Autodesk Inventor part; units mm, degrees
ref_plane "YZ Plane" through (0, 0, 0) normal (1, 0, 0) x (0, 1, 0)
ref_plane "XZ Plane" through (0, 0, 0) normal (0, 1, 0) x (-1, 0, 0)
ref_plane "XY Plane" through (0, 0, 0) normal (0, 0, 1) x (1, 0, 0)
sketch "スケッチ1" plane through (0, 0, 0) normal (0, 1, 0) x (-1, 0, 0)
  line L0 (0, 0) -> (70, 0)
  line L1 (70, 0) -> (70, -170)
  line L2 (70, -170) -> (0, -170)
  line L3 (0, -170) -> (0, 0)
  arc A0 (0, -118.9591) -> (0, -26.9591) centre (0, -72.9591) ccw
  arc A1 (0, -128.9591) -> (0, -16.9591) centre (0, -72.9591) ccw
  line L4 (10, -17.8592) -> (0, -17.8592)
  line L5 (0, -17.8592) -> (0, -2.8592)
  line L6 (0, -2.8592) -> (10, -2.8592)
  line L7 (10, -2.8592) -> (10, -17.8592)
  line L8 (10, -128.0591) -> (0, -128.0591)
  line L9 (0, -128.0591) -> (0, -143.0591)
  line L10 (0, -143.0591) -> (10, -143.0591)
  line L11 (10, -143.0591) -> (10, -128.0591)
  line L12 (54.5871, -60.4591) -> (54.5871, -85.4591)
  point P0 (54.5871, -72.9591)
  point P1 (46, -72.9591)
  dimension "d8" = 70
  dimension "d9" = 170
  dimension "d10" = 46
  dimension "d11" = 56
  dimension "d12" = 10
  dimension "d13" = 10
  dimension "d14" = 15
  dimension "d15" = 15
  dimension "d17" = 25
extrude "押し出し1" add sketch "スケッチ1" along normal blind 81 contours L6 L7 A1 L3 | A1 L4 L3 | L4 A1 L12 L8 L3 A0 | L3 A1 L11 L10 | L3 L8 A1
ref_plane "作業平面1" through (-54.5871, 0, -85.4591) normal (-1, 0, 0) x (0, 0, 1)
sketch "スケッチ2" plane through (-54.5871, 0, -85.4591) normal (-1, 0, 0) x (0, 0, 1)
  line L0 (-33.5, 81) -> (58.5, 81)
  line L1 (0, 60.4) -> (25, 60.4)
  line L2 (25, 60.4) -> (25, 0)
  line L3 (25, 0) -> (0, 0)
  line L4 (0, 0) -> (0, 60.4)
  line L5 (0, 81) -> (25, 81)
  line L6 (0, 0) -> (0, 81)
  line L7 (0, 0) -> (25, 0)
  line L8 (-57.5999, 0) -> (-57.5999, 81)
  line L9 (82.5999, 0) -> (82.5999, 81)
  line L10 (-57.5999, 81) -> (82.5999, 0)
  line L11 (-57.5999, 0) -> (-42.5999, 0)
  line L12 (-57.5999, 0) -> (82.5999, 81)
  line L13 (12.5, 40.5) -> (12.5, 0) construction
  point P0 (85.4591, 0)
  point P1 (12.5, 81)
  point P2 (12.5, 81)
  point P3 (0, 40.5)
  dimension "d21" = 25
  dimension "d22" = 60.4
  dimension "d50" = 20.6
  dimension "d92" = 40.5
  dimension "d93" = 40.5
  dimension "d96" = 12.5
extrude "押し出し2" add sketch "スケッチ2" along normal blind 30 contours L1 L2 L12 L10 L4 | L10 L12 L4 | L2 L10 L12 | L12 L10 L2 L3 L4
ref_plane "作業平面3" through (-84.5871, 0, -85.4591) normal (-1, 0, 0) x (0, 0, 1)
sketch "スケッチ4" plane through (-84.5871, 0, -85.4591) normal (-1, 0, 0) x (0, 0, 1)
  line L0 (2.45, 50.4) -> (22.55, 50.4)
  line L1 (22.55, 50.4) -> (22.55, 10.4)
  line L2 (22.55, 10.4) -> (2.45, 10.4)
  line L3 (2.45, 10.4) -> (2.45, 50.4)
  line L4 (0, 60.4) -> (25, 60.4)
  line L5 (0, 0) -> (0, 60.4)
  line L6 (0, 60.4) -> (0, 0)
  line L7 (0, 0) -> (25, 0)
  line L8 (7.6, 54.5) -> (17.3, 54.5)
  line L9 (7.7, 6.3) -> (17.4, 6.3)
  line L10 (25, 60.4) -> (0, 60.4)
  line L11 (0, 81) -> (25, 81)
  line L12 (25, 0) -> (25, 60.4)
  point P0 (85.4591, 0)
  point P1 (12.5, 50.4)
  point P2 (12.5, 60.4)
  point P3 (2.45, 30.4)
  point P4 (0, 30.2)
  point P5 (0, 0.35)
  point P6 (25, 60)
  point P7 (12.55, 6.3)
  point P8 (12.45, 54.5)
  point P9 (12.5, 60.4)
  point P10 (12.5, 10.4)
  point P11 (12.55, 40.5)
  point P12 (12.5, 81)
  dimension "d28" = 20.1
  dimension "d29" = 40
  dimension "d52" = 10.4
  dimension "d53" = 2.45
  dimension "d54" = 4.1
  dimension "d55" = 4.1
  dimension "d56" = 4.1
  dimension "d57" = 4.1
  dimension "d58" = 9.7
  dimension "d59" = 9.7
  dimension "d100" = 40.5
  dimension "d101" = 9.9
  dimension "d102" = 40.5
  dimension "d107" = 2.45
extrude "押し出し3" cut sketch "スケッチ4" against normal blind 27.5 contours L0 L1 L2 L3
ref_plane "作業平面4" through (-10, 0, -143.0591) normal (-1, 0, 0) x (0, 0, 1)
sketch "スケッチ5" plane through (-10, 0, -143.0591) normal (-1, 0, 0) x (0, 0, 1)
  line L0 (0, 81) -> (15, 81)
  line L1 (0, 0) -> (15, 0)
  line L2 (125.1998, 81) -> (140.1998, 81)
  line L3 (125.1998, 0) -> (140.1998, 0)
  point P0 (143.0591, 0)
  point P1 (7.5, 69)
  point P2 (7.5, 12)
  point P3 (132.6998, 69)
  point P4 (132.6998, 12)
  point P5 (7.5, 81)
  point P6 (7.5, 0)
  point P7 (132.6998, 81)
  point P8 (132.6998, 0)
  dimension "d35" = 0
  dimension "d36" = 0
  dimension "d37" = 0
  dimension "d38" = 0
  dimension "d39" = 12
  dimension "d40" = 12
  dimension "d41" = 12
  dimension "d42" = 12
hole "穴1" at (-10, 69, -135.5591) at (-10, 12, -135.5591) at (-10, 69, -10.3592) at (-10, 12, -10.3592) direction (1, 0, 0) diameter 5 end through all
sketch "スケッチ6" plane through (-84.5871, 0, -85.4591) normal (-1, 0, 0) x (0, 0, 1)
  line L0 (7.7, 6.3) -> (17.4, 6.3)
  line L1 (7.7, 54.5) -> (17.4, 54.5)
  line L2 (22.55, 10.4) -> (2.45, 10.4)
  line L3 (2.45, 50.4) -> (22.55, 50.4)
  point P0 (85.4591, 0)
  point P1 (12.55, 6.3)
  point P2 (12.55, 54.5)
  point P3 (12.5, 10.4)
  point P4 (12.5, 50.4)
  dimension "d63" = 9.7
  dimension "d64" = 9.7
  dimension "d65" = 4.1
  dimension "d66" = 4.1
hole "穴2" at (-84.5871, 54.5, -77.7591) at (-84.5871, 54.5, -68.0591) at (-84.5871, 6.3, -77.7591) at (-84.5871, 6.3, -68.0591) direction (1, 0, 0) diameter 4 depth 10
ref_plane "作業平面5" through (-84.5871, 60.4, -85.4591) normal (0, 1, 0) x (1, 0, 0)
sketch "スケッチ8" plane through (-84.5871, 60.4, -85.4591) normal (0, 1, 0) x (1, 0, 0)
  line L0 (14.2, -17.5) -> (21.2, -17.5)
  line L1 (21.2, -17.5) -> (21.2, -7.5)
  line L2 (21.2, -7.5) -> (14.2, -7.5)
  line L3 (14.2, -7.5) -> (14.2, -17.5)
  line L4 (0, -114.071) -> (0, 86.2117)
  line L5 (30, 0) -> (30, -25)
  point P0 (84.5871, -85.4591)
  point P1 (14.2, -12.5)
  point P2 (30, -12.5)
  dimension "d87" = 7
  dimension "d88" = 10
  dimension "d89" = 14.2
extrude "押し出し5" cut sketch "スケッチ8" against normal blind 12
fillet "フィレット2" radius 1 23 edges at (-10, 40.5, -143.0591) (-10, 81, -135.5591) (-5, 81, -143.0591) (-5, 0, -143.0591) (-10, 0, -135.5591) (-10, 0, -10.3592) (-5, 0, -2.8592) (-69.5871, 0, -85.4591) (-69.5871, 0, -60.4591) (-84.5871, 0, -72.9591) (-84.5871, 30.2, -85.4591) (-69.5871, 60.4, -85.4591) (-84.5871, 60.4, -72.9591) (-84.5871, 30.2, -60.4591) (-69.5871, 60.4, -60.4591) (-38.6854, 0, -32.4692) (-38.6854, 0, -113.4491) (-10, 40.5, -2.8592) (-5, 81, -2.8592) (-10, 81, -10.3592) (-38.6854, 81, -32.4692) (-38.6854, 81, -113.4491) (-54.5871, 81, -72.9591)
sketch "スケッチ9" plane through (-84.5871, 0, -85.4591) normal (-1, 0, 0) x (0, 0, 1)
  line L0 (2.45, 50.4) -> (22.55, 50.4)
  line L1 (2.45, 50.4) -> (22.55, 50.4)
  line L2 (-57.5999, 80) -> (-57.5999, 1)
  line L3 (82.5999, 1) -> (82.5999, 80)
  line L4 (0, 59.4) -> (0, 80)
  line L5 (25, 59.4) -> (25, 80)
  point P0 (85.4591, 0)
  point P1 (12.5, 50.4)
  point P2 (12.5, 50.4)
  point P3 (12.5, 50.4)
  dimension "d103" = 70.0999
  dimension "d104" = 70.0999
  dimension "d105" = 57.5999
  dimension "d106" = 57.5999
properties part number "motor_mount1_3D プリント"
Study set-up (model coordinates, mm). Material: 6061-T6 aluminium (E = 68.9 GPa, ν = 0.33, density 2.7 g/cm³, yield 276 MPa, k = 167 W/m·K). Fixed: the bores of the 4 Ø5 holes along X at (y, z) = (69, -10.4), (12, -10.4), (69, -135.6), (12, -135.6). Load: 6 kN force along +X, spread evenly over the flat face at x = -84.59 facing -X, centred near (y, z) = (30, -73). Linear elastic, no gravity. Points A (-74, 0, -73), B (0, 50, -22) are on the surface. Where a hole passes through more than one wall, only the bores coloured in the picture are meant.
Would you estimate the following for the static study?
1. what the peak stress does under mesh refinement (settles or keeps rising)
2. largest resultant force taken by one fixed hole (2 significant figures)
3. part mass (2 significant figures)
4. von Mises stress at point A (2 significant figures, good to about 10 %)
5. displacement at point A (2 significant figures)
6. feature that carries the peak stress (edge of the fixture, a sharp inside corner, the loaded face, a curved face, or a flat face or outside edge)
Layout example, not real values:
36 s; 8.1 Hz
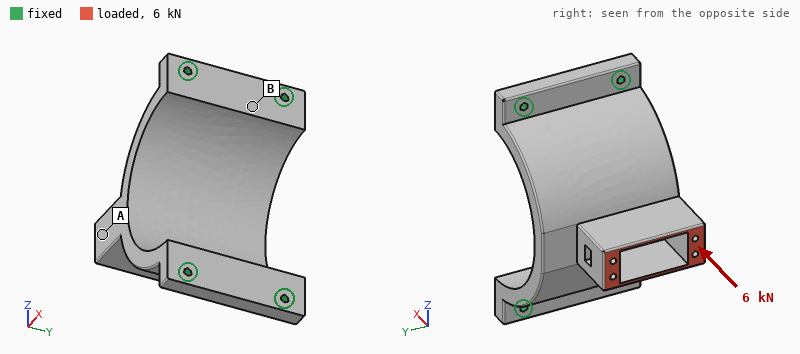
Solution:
keeps rising; 2.7 kN; 460 g; 8.8 MPa; 38 µm; edge of the fixture
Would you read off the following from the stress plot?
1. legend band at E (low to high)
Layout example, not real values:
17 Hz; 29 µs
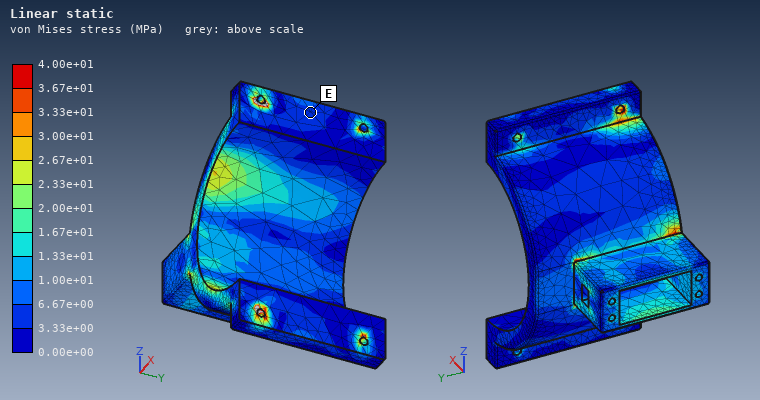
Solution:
3.33e+00 to 6.67e+00 MPa
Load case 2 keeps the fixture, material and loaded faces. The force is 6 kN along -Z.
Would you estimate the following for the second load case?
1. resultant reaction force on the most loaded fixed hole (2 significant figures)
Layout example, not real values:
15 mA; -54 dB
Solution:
2.9 kN
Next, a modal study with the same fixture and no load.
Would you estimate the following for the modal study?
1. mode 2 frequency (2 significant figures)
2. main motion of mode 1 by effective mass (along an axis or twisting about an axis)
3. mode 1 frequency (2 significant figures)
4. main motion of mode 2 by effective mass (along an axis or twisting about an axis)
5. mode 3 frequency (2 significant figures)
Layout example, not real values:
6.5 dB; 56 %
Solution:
3900 Hz; along Z; 3400 Hz; along Y; 5700 Hz
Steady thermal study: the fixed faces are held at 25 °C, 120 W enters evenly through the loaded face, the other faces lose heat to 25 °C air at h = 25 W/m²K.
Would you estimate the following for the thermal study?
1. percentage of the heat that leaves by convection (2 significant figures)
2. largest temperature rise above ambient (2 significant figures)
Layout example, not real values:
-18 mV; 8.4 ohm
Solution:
21 %; 70 K
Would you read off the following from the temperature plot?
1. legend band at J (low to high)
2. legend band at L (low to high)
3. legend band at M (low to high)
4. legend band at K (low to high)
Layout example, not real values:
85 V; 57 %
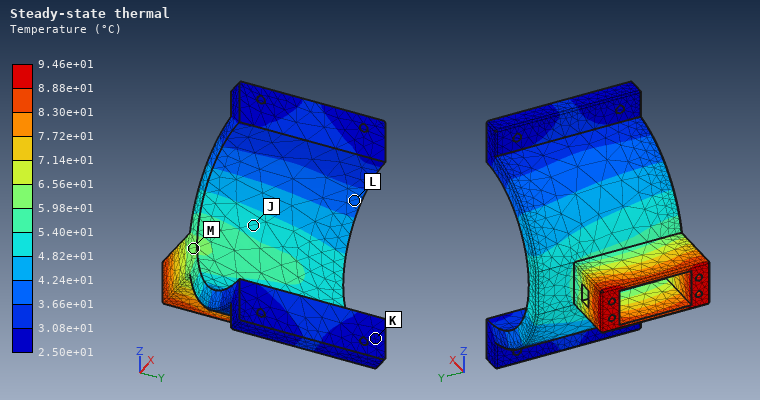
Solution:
4.82e+01 to 5.40e+01 °C; 3.66e+01 to 4.24e+01 °C; 5.98e+01 to 6.56e+01 °C; 2.50e+01 to 3.08e+01 °C
